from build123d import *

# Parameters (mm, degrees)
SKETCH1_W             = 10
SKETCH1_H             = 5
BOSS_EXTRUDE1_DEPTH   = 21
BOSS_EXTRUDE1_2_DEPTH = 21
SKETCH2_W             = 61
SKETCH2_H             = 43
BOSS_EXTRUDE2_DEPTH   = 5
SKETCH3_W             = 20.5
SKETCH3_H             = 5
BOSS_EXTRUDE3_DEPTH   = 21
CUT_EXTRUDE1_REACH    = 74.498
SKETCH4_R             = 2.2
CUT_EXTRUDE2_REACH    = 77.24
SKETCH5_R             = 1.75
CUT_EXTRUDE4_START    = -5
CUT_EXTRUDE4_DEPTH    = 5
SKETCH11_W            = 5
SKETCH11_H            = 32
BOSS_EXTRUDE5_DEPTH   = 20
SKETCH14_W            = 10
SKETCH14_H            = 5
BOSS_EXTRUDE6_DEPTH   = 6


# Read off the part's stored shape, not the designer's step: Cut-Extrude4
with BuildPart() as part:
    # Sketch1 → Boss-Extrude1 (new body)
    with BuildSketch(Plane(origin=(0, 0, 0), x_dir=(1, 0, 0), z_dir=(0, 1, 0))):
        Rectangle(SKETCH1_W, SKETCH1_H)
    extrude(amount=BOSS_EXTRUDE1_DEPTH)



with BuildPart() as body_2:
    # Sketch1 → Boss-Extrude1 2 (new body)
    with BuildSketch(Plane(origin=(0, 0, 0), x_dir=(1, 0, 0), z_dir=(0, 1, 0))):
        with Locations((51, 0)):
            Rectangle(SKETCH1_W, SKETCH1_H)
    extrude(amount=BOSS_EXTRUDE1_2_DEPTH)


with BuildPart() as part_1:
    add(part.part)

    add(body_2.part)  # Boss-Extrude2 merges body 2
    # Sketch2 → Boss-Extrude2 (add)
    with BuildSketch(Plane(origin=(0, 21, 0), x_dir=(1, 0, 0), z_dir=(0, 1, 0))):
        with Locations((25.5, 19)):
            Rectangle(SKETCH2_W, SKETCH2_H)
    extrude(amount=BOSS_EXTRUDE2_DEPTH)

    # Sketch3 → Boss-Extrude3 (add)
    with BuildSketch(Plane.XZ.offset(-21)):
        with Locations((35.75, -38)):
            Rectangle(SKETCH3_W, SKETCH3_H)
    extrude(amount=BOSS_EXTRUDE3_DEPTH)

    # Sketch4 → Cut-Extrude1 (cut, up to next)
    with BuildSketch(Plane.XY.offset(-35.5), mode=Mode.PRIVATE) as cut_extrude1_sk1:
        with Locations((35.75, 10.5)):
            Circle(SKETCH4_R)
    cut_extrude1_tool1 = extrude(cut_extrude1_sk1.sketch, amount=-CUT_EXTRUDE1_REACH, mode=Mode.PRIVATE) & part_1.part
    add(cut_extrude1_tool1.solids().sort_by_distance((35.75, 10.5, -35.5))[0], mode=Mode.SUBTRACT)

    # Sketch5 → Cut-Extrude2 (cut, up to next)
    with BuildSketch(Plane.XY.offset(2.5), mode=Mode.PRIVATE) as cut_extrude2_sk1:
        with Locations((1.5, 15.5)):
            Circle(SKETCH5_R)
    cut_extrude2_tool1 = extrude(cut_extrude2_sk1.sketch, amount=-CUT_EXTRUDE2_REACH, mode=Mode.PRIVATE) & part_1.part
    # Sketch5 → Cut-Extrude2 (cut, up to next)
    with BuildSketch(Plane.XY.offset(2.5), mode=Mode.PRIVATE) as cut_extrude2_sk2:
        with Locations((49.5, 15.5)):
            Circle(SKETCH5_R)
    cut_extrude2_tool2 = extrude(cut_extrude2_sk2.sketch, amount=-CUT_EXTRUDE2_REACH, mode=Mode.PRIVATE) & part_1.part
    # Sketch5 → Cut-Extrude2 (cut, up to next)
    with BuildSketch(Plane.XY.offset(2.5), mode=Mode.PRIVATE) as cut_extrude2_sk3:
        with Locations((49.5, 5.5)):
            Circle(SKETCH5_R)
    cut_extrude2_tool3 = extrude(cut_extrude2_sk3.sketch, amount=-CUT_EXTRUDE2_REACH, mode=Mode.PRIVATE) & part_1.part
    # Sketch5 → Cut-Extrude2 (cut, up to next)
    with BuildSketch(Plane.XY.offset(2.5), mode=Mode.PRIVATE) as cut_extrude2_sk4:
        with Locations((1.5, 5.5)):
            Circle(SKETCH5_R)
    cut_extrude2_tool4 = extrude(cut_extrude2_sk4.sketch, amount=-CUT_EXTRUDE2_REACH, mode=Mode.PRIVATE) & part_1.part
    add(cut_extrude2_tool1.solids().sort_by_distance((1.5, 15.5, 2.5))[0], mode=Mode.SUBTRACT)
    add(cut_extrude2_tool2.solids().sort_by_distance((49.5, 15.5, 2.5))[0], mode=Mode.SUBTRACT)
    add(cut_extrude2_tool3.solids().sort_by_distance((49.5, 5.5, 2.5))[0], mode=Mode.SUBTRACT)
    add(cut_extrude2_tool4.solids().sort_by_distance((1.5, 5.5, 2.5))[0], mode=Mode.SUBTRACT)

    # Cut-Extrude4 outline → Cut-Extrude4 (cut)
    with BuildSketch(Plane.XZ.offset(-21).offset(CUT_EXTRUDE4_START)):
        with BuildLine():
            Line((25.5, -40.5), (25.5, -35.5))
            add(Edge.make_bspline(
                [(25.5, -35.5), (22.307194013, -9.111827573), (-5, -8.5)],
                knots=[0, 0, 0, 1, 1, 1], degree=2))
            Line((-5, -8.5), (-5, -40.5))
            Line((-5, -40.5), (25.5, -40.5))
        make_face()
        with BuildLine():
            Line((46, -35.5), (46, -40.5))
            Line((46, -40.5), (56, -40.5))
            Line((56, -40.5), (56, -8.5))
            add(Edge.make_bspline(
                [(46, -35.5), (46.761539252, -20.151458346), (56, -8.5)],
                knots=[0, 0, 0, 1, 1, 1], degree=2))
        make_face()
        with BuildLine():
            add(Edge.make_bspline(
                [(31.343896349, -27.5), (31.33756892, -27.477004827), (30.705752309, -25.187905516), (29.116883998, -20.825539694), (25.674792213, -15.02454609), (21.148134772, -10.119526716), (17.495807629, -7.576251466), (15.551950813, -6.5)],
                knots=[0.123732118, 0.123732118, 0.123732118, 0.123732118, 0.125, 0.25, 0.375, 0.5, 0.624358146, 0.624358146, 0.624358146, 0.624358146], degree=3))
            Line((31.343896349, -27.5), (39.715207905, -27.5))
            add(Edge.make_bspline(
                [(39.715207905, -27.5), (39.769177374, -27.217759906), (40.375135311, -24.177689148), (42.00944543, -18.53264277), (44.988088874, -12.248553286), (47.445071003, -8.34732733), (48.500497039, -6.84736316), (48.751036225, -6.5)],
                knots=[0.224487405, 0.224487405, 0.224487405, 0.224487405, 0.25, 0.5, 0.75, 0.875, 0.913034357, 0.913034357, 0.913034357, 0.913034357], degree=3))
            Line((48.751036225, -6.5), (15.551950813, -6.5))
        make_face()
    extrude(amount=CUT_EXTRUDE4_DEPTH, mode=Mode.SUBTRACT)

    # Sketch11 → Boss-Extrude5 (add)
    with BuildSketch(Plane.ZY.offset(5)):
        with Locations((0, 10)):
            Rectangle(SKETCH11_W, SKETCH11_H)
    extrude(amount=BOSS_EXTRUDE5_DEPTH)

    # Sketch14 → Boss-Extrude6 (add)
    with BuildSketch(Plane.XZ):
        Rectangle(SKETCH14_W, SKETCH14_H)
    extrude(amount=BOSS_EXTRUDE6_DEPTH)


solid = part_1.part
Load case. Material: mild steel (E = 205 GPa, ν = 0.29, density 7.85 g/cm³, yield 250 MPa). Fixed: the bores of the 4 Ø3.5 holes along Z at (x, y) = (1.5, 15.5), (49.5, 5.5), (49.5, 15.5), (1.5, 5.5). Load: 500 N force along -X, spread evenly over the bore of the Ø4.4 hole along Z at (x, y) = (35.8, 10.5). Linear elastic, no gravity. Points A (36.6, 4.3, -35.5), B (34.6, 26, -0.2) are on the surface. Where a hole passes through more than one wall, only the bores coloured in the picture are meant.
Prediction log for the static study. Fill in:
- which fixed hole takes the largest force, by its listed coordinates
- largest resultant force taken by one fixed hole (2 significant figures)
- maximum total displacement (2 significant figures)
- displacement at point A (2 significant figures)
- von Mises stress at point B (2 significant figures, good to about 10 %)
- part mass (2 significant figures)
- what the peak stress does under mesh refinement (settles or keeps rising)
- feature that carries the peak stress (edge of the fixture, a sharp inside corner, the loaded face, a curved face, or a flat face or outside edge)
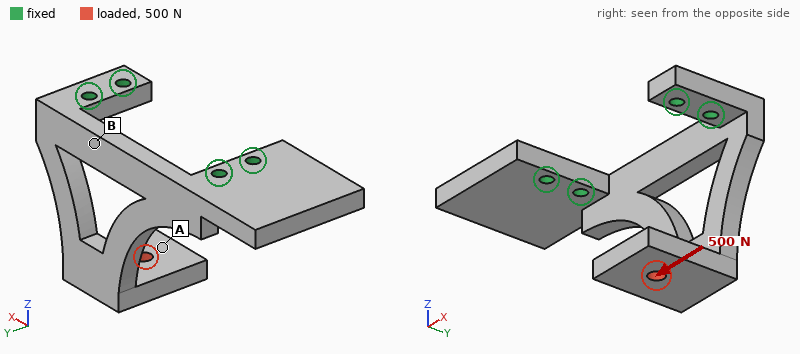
(1.5, 15.5)
660 N
0.12 mm
0.096 mm
26 MPa
110 g
keeps rising
edge of the fixture
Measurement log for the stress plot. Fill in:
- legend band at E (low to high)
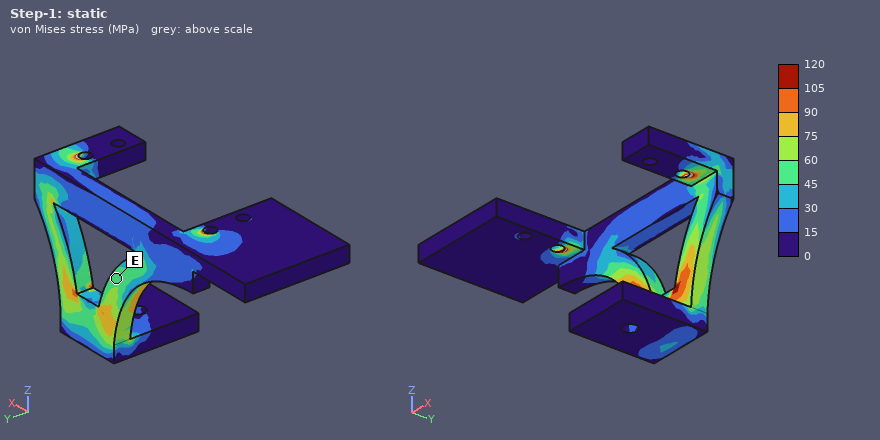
45 to 60 MPa
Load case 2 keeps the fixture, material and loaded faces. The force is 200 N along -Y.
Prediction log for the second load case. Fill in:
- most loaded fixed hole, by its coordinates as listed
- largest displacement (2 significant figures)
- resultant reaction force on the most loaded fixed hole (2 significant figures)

(49.5, 15.5)
0.23 mm
170 N
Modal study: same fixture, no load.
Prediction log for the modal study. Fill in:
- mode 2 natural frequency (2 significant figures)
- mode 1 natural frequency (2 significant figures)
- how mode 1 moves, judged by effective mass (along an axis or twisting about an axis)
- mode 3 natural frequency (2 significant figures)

2800 Hz
990 Hz
along Y
3700 Hz
